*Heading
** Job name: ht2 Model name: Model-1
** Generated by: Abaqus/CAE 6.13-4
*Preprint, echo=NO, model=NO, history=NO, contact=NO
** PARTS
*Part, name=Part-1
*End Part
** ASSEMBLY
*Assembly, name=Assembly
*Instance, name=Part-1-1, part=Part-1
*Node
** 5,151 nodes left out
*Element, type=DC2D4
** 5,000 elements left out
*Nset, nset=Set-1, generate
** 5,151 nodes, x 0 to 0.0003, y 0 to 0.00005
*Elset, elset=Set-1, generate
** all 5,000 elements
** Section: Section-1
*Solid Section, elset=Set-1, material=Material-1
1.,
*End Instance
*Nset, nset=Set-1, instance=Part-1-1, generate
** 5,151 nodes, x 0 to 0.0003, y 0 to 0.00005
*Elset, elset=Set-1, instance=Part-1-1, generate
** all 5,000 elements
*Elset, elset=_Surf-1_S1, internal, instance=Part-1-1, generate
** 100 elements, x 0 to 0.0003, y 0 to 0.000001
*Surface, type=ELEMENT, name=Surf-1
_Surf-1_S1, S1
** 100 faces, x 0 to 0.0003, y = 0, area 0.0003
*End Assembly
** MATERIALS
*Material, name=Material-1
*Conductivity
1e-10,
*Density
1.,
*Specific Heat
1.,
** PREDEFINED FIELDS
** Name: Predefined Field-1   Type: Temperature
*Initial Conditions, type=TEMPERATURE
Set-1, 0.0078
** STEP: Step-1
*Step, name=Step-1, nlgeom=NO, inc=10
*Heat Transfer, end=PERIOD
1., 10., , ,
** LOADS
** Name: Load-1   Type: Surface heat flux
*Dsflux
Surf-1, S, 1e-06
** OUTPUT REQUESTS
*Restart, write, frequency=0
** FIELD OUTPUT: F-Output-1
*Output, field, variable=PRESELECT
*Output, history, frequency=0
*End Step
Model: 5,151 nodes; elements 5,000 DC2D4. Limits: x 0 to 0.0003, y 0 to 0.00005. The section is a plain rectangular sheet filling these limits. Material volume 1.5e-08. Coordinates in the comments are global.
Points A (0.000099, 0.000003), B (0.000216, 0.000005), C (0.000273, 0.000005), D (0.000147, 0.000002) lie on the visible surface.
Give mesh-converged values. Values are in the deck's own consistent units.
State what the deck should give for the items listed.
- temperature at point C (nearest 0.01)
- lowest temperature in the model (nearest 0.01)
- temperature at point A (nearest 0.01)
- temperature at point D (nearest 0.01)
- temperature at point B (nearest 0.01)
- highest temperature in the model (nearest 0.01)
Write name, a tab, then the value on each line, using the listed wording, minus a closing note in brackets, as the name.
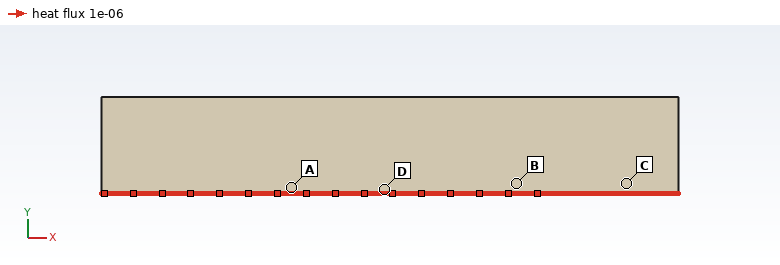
temperature at point C	0.32
lowest temperature in the model	0.13
temperature at point A	0.34
temperature at point D	0.35
temperature at point B	0.32
highest temperature in the model	0.37
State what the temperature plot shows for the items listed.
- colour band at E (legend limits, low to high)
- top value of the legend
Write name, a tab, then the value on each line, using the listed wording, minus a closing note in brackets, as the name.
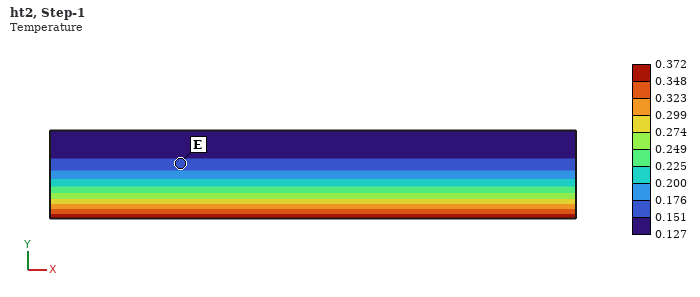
colour band at E	0.151 to 0.176
top value of the legend	0.372
